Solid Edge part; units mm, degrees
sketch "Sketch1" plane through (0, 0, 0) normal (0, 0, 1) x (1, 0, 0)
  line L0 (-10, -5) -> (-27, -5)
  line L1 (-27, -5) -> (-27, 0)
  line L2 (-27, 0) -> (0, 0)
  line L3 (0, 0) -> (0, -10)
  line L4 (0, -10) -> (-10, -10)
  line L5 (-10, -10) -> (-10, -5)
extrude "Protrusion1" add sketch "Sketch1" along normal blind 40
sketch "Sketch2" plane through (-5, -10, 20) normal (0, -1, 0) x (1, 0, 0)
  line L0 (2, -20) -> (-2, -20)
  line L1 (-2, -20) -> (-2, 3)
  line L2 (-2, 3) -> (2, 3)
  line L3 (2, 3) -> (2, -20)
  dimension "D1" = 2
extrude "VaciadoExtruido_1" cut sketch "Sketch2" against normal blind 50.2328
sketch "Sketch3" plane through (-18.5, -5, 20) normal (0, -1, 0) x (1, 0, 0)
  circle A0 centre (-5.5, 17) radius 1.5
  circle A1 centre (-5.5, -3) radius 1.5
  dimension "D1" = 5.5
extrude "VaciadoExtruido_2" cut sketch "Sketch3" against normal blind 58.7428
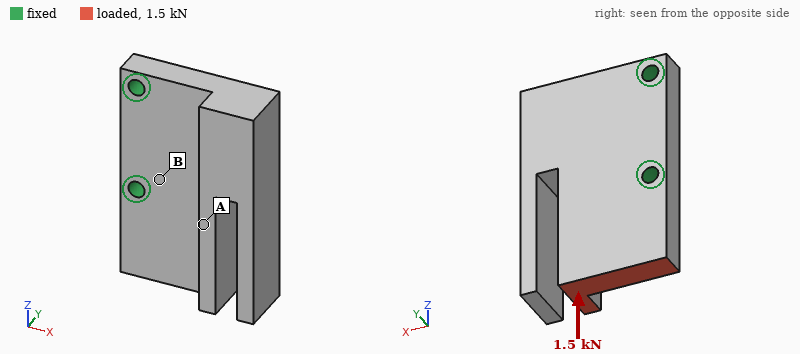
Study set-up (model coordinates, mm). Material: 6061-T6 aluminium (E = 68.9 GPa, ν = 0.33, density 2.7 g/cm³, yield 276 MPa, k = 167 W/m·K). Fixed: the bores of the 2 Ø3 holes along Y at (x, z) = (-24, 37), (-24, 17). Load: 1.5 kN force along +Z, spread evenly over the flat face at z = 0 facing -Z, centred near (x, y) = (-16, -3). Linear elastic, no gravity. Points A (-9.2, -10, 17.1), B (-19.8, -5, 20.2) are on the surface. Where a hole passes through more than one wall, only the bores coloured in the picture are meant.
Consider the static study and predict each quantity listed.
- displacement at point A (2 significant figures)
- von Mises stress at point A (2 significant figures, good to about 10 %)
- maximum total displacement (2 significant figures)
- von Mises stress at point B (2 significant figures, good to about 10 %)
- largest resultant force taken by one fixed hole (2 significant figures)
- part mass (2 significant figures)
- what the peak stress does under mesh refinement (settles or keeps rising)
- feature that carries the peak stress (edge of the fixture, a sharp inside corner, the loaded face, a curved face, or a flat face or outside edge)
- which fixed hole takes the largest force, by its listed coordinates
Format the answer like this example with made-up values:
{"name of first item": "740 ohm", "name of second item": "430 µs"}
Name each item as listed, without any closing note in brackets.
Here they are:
{"displacement at point A": "9.0 µm", "von Mises stress at point A": "8.2 MPa", "maximum total displacement": "15 µm", "von Mises stress at point B": "22 MPa", "largest resultant force taken by one fixed hole": "1.1 kN", "part mass": "17 g", "what the peak stress does under mesh refinement": "keeps rising", "feature that carries the peak stress": "edge of the fixture", "which fixed hole takes the largest force, by its listed coordinates": "(-24, 17)"}
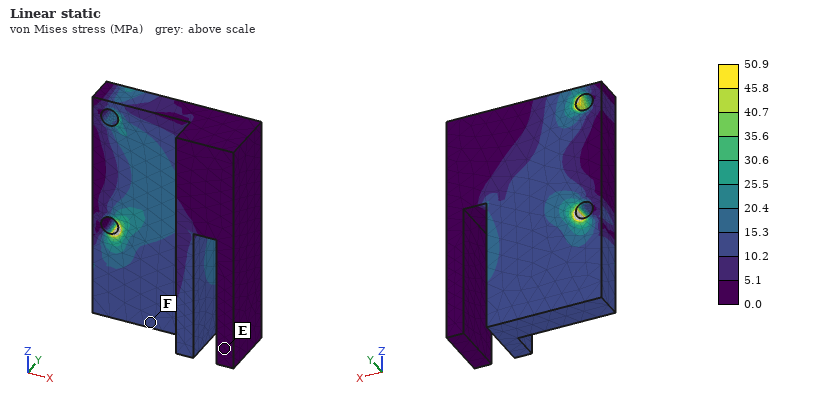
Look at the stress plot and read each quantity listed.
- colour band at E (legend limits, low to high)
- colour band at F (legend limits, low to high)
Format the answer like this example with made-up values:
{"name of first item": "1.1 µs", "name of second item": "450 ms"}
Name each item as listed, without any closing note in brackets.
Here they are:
{"colour band at E": "0.0 to 5.1 MPa", "colour band at F": "10.2 to 15.3 MPa"}
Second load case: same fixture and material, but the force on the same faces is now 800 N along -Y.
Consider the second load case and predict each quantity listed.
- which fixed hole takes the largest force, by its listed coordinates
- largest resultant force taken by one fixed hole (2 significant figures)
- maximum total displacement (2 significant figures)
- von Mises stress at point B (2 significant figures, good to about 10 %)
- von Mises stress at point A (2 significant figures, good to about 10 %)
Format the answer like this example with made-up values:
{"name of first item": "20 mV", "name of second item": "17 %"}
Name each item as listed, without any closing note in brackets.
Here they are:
{"which fixed hole takes the largest force, by its listed coordinates": "(-24, 17)", "largest resultant force taken by one fixed hole": "1.2 kN", "maximum total displacement": "0.15 mm", "von Mises stress at point B": "64 MPa", "von Mises stress at point A": "73 MPa"}
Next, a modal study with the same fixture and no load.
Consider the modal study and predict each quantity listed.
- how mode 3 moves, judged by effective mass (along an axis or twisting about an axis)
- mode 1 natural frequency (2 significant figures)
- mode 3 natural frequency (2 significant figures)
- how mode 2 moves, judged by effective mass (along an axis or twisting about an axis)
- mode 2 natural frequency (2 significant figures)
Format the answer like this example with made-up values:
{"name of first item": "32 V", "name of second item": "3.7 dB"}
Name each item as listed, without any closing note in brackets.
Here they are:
{"how mode 3 moves, judged by effective mass": "twisting about X", "mode 1 natural frequency": "3900 Hz", "mode 3 natural frequency": "7500 Hz", "how mode 2 moves, judged by effective mass": "along Y", "mode 2 natural frequency": "4300 Hz"}
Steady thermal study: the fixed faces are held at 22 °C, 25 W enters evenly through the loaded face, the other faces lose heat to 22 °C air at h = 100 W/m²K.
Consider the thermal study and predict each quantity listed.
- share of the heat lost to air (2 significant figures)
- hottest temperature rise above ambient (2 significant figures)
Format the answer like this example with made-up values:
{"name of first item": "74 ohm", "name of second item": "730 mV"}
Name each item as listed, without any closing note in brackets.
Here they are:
{"share of the heat lost to air": "11 %", "hottest temperature rise above ambient": "28 K"}
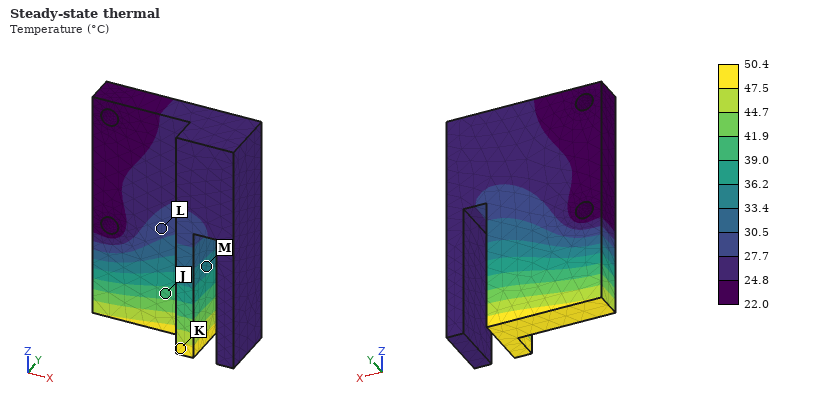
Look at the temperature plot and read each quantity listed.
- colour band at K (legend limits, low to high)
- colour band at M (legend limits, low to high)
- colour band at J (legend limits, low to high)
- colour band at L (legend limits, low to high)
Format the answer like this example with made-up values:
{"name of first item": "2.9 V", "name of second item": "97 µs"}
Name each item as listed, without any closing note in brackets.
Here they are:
{"colour band at K": "47.5 to 50.4 °C", "colour band at M": "33.4 to 36.2 °C", "colour band at J": "39.0 to 41.9 °C", "colour band at L": "27.7 to 30.5 °C"}
